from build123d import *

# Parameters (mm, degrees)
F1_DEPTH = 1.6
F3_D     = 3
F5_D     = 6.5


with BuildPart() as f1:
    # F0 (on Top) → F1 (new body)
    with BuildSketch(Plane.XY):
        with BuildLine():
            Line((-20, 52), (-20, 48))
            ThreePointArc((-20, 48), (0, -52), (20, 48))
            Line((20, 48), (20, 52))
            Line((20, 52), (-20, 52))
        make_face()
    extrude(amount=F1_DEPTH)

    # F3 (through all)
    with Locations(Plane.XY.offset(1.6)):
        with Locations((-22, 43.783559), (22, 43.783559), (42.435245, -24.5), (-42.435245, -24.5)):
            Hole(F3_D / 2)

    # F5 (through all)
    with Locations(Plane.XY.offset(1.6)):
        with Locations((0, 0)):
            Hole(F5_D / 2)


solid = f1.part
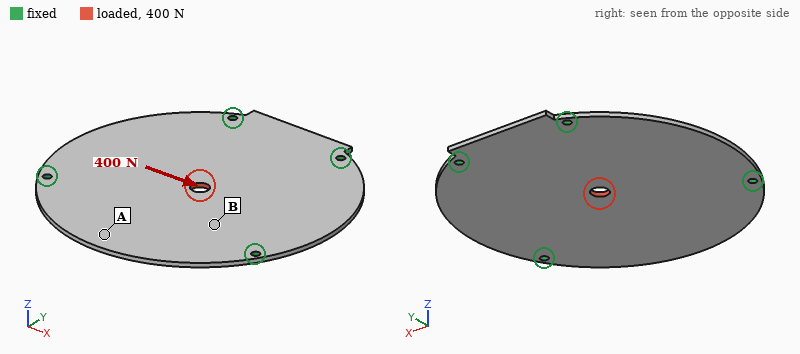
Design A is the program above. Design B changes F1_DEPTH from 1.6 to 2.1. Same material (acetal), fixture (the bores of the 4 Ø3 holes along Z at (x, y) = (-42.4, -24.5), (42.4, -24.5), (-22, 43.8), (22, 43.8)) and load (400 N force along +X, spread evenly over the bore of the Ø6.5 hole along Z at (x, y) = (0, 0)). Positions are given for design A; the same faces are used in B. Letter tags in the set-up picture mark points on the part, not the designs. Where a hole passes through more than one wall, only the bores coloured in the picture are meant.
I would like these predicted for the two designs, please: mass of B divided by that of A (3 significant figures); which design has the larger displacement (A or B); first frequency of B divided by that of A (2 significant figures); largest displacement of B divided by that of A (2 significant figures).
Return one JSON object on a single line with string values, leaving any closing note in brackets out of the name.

{"mass of B divided by that of A": "1.31", "which design has the larger displacement": "A", "first frequency of B divided by that of A": "1.3", "largest displacement of B divided by that of A": "0.76"}
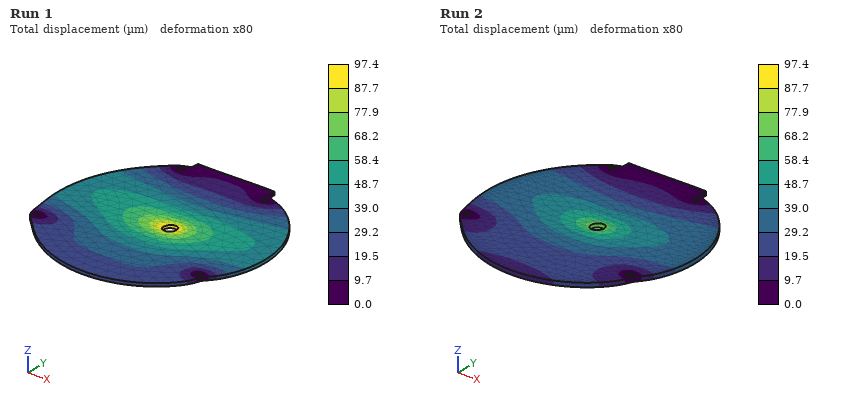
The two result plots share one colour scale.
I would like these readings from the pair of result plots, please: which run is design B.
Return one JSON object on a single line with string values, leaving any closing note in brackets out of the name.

{"which run is design B": "Run 2"}
